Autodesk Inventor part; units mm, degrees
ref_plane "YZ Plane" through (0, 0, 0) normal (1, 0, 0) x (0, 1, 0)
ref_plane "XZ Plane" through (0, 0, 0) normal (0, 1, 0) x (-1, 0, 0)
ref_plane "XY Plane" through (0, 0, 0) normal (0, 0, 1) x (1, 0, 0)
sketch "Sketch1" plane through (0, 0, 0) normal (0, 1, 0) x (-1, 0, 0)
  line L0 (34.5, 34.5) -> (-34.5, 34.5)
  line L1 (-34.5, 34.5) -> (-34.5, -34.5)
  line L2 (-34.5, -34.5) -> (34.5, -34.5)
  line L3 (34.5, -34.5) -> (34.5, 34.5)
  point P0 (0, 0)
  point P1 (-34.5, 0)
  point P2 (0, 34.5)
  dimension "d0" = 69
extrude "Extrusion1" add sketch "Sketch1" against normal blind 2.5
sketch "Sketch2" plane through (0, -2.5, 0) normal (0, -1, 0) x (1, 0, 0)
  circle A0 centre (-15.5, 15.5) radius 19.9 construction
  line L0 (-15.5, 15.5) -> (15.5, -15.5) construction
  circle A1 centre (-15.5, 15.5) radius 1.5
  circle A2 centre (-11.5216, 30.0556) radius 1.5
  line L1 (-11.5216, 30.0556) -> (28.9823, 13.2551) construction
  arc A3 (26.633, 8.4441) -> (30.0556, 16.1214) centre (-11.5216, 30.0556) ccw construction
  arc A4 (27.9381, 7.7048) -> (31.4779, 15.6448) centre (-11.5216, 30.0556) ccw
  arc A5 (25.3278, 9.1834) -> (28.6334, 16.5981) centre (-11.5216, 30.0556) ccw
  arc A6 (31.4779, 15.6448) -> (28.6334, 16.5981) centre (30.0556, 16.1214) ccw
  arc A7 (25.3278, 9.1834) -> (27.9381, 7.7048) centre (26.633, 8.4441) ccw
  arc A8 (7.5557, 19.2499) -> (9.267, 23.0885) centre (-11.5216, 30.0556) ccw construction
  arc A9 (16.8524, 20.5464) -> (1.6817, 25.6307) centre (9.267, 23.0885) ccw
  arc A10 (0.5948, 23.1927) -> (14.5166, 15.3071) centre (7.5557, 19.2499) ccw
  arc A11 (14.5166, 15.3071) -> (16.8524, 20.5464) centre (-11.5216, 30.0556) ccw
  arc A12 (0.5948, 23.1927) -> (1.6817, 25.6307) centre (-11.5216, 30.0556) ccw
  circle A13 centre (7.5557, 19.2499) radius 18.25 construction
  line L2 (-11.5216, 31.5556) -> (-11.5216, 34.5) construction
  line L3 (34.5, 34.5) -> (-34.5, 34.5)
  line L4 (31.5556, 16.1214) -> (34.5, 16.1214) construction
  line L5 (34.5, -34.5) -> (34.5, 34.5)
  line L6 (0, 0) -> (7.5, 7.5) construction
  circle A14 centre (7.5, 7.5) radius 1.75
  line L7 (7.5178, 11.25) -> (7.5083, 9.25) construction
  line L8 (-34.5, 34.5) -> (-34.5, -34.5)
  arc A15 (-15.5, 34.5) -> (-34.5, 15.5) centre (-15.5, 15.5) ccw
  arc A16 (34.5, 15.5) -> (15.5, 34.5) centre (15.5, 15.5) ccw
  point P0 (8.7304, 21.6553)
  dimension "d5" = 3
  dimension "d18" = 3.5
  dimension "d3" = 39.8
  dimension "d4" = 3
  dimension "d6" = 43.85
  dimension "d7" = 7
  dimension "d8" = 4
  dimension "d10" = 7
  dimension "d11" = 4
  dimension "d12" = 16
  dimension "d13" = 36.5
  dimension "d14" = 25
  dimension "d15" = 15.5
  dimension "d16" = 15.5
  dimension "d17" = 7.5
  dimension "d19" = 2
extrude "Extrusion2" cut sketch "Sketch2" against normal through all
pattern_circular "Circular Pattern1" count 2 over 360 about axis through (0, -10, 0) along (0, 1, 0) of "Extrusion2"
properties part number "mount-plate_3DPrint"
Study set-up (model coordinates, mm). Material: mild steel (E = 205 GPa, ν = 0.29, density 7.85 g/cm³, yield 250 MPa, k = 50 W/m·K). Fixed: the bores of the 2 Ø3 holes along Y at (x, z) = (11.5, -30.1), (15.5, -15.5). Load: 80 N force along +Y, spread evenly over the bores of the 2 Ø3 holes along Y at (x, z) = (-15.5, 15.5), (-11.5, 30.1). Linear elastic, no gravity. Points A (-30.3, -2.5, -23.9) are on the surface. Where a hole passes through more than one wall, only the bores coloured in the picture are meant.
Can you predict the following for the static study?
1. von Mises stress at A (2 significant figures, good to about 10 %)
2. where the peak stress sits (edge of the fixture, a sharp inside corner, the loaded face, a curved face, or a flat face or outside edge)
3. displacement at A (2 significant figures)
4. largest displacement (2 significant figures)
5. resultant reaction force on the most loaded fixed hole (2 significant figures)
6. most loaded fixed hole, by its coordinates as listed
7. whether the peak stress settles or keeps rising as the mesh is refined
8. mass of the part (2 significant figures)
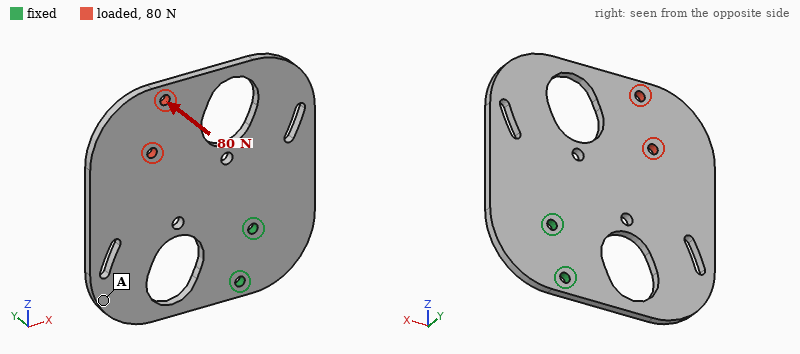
18 MPa
edge of the fixture
0.11 mm
0.44 mm
160 N
(15.5, -15.5)
keeps rising
75 g
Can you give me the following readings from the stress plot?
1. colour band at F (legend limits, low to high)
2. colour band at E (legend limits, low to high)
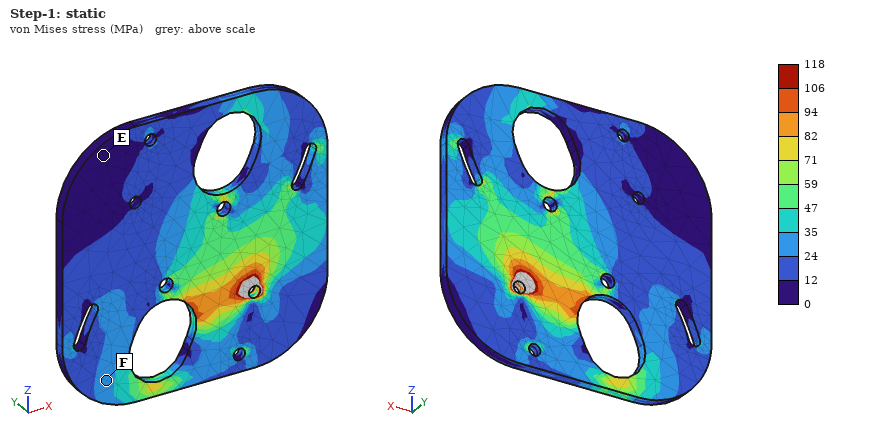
24 to 35 MPa
0 to 12 MPa
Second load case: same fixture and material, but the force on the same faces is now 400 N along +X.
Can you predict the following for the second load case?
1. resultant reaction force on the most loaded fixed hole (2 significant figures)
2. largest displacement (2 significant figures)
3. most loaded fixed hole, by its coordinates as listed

1.3 kN
24 µm
(15.5, -15.5)
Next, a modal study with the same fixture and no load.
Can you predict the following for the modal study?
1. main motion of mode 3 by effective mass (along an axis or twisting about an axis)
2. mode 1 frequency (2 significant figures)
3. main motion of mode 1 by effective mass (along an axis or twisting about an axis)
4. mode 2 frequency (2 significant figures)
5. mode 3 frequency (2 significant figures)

along Y
510 Hz
along Y
980 Hz
1900 Hz
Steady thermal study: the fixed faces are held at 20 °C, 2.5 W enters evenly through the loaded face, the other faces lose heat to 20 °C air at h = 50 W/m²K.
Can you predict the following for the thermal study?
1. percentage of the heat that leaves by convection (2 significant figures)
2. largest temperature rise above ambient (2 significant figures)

77 %
15 K
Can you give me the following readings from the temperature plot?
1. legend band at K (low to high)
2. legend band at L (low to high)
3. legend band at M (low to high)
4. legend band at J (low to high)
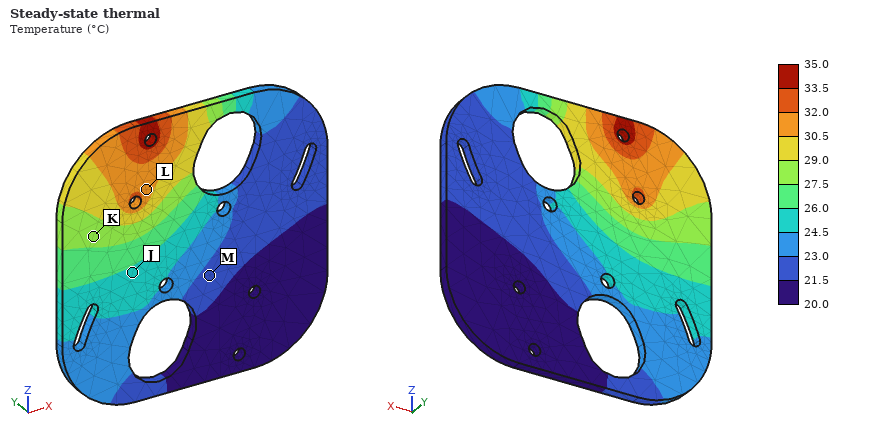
27.5 to 29.0 °C
30.5 to 32.0 °C
21.5 to 23.0 °C
24.5 to 26.0 °C
